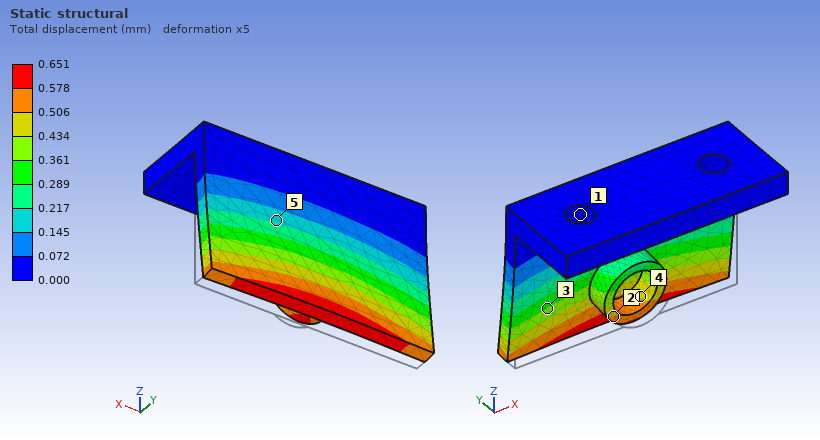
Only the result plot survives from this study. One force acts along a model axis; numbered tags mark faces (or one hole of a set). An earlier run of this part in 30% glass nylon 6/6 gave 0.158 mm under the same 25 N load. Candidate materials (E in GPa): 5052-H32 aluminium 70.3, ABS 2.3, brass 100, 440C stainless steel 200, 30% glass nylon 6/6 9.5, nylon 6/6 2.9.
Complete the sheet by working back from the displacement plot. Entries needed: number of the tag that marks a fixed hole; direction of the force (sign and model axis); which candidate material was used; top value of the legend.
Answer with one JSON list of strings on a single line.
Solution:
["1", "+Y", "ABS", "0.651 mm"]
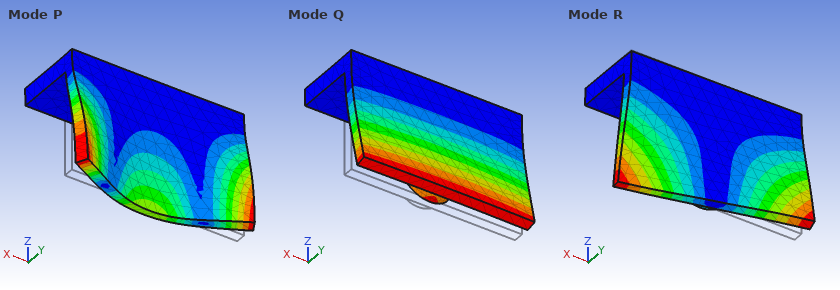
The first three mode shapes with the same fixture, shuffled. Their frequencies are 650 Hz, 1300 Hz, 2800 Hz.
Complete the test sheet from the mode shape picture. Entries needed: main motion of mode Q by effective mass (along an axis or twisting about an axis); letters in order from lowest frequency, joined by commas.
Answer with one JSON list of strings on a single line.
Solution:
["along Y", "Q, R, P"]
